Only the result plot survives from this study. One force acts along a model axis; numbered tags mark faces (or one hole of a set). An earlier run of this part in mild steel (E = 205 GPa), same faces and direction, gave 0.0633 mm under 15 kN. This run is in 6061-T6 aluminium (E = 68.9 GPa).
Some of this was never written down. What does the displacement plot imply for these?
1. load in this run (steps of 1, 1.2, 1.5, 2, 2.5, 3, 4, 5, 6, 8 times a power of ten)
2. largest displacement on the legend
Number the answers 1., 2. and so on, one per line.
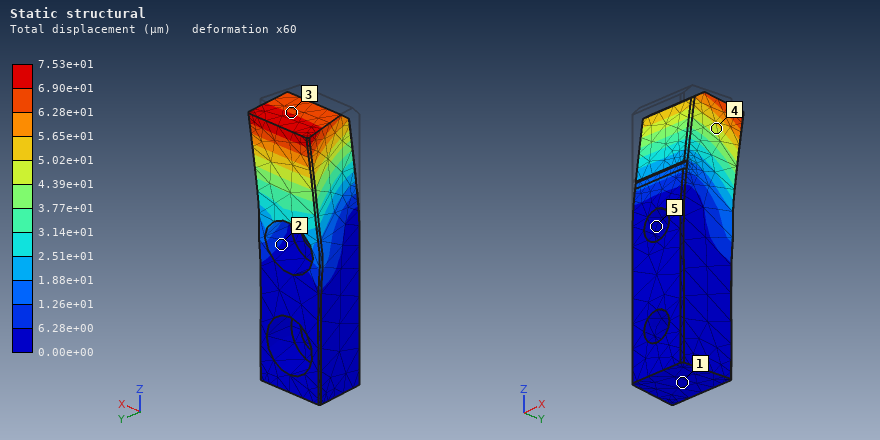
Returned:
1. 6 kN
2. 7.53e+01 µm
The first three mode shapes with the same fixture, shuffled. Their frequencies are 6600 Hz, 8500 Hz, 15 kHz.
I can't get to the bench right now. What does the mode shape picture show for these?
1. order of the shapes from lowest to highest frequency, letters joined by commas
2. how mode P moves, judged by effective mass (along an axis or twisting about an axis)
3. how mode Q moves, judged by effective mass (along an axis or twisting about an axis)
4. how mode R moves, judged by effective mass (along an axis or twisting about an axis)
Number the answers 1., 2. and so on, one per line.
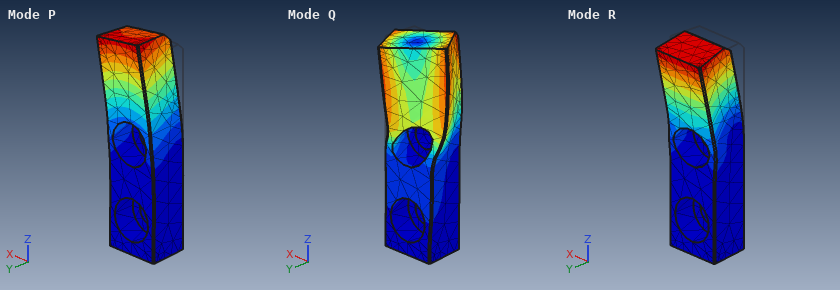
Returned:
1. R, P, Q
2. along X
3. twisting about Z
4. along Y
